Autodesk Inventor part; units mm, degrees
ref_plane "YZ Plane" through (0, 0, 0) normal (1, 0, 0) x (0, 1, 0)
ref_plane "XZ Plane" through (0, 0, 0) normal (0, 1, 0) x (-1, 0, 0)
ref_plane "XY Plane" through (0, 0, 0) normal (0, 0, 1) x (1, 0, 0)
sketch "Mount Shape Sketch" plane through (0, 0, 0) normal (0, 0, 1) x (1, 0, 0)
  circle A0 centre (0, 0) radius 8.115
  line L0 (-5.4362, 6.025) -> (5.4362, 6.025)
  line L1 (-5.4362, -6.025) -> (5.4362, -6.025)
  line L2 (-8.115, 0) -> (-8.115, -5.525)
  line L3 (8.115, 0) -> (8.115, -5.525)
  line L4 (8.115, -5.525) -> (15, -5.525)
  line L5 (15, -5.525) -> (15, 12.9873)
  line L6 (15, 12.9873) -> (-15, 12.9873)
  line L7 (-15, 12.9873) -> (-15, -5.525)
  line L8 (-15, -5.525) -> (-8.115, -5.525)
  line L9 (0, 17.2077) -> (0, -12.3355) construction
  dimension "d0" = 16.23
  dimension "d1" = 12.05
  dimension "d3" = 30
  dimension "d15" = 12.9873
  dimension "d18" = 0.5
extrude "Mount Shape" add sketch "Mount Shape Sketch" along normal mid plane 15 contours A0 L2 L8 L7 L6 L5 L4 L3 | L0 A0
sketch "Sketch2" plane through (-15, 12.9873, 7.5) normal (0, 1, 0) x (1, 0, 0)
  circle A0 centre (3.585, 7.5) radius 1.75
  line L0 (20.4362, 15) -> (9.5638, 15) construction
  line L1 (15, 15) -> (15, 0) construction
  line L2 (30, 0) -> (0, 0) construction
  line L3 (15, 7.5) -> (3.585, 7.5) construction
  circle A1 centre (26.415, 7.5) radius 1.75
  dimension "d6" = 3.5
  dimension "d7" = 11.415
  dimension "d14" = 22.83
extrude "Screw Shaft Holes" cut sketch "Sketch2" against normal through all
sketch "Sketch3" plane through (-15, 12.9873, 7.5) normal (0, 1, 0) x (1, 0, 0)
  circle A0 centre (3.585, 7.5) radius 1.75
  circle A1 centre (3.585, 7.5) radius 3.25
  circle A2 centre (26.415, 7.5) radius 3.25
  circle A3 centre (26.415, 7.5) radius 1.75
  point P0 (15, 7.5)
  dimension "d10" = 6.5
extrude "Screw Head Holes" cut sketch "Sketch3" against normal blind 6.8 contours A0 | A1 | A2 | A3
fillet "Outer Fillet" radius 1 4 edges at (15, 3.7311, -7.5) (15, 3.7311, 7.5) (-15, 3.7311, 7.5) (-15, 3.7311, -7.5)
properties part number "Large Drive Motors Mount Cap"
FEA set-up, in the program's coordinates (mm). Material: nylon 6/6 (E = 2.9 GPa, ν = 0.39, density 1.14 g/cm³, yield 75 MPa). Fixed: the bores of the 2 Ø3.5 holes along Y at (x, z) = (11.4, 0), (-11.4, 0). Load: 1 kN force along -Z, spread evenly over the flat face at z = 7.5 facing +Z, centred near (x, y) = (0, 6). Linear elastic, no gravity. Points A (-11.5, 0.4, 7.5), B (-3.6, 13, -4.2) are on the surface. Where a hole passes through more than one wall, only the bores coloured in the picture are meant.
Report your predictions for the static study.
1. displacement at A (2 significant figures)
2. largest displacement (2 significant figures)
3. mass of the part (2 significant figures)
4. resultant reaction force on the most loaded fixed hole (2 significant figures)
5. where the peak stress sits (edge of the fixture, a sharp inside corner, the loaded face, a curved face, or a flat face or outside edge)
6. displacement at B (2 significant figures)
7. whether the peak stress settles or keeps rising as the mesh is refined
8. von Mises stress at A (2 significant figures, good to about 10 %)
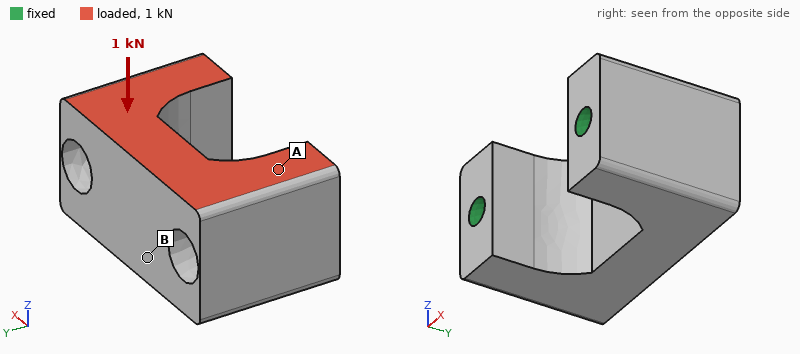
19 µm
92 µm
5.7 g
500 N
edge of the fixture
72 µm
keeps rising
6.0 MPa
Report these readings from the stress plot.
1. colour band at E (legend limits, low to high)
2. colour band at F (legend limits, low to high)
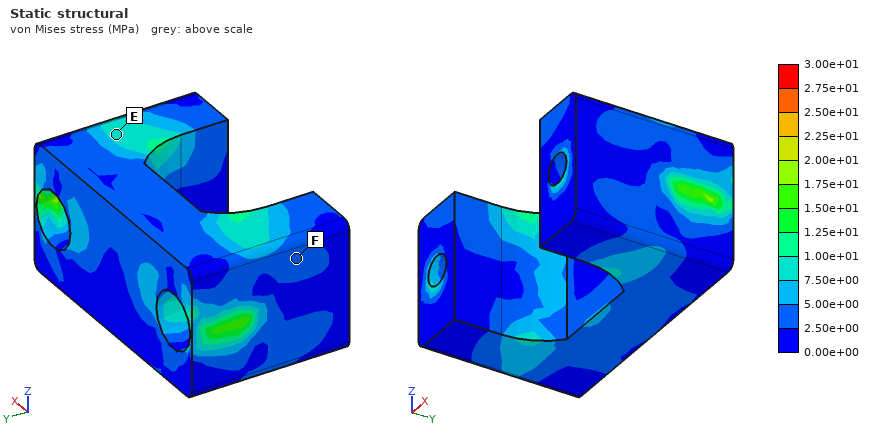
7.50e+00 to 1.00e+01 MPa
2.50e+00 to 5.00e+00 MPa
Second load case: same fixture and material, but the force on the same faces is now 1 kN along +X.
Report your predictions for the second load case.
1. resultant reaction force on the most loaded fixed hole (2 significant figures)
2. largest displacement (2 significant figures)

550 N
85 µm
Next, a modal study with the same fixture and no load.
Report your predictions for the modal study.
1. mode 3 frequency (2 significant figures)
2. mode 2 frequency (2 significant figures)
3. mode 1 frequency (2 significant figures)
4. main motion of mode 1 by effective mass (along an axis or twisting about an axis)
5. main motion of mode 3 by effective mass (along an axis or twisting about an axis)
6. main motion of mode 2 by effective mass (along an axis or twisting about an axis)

14 kHz
13 kHz
8800 Hz
along Z
twisting about Y
along X
